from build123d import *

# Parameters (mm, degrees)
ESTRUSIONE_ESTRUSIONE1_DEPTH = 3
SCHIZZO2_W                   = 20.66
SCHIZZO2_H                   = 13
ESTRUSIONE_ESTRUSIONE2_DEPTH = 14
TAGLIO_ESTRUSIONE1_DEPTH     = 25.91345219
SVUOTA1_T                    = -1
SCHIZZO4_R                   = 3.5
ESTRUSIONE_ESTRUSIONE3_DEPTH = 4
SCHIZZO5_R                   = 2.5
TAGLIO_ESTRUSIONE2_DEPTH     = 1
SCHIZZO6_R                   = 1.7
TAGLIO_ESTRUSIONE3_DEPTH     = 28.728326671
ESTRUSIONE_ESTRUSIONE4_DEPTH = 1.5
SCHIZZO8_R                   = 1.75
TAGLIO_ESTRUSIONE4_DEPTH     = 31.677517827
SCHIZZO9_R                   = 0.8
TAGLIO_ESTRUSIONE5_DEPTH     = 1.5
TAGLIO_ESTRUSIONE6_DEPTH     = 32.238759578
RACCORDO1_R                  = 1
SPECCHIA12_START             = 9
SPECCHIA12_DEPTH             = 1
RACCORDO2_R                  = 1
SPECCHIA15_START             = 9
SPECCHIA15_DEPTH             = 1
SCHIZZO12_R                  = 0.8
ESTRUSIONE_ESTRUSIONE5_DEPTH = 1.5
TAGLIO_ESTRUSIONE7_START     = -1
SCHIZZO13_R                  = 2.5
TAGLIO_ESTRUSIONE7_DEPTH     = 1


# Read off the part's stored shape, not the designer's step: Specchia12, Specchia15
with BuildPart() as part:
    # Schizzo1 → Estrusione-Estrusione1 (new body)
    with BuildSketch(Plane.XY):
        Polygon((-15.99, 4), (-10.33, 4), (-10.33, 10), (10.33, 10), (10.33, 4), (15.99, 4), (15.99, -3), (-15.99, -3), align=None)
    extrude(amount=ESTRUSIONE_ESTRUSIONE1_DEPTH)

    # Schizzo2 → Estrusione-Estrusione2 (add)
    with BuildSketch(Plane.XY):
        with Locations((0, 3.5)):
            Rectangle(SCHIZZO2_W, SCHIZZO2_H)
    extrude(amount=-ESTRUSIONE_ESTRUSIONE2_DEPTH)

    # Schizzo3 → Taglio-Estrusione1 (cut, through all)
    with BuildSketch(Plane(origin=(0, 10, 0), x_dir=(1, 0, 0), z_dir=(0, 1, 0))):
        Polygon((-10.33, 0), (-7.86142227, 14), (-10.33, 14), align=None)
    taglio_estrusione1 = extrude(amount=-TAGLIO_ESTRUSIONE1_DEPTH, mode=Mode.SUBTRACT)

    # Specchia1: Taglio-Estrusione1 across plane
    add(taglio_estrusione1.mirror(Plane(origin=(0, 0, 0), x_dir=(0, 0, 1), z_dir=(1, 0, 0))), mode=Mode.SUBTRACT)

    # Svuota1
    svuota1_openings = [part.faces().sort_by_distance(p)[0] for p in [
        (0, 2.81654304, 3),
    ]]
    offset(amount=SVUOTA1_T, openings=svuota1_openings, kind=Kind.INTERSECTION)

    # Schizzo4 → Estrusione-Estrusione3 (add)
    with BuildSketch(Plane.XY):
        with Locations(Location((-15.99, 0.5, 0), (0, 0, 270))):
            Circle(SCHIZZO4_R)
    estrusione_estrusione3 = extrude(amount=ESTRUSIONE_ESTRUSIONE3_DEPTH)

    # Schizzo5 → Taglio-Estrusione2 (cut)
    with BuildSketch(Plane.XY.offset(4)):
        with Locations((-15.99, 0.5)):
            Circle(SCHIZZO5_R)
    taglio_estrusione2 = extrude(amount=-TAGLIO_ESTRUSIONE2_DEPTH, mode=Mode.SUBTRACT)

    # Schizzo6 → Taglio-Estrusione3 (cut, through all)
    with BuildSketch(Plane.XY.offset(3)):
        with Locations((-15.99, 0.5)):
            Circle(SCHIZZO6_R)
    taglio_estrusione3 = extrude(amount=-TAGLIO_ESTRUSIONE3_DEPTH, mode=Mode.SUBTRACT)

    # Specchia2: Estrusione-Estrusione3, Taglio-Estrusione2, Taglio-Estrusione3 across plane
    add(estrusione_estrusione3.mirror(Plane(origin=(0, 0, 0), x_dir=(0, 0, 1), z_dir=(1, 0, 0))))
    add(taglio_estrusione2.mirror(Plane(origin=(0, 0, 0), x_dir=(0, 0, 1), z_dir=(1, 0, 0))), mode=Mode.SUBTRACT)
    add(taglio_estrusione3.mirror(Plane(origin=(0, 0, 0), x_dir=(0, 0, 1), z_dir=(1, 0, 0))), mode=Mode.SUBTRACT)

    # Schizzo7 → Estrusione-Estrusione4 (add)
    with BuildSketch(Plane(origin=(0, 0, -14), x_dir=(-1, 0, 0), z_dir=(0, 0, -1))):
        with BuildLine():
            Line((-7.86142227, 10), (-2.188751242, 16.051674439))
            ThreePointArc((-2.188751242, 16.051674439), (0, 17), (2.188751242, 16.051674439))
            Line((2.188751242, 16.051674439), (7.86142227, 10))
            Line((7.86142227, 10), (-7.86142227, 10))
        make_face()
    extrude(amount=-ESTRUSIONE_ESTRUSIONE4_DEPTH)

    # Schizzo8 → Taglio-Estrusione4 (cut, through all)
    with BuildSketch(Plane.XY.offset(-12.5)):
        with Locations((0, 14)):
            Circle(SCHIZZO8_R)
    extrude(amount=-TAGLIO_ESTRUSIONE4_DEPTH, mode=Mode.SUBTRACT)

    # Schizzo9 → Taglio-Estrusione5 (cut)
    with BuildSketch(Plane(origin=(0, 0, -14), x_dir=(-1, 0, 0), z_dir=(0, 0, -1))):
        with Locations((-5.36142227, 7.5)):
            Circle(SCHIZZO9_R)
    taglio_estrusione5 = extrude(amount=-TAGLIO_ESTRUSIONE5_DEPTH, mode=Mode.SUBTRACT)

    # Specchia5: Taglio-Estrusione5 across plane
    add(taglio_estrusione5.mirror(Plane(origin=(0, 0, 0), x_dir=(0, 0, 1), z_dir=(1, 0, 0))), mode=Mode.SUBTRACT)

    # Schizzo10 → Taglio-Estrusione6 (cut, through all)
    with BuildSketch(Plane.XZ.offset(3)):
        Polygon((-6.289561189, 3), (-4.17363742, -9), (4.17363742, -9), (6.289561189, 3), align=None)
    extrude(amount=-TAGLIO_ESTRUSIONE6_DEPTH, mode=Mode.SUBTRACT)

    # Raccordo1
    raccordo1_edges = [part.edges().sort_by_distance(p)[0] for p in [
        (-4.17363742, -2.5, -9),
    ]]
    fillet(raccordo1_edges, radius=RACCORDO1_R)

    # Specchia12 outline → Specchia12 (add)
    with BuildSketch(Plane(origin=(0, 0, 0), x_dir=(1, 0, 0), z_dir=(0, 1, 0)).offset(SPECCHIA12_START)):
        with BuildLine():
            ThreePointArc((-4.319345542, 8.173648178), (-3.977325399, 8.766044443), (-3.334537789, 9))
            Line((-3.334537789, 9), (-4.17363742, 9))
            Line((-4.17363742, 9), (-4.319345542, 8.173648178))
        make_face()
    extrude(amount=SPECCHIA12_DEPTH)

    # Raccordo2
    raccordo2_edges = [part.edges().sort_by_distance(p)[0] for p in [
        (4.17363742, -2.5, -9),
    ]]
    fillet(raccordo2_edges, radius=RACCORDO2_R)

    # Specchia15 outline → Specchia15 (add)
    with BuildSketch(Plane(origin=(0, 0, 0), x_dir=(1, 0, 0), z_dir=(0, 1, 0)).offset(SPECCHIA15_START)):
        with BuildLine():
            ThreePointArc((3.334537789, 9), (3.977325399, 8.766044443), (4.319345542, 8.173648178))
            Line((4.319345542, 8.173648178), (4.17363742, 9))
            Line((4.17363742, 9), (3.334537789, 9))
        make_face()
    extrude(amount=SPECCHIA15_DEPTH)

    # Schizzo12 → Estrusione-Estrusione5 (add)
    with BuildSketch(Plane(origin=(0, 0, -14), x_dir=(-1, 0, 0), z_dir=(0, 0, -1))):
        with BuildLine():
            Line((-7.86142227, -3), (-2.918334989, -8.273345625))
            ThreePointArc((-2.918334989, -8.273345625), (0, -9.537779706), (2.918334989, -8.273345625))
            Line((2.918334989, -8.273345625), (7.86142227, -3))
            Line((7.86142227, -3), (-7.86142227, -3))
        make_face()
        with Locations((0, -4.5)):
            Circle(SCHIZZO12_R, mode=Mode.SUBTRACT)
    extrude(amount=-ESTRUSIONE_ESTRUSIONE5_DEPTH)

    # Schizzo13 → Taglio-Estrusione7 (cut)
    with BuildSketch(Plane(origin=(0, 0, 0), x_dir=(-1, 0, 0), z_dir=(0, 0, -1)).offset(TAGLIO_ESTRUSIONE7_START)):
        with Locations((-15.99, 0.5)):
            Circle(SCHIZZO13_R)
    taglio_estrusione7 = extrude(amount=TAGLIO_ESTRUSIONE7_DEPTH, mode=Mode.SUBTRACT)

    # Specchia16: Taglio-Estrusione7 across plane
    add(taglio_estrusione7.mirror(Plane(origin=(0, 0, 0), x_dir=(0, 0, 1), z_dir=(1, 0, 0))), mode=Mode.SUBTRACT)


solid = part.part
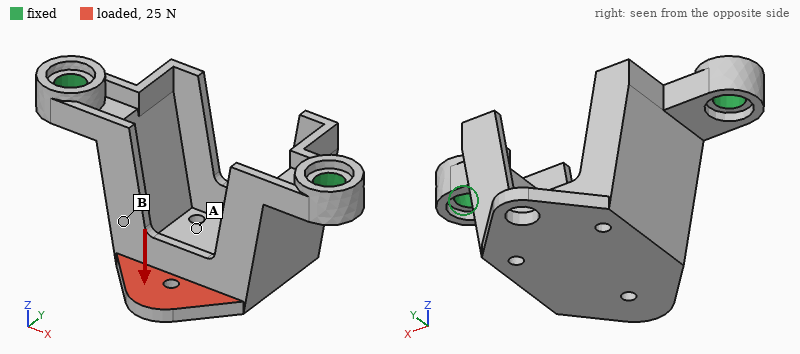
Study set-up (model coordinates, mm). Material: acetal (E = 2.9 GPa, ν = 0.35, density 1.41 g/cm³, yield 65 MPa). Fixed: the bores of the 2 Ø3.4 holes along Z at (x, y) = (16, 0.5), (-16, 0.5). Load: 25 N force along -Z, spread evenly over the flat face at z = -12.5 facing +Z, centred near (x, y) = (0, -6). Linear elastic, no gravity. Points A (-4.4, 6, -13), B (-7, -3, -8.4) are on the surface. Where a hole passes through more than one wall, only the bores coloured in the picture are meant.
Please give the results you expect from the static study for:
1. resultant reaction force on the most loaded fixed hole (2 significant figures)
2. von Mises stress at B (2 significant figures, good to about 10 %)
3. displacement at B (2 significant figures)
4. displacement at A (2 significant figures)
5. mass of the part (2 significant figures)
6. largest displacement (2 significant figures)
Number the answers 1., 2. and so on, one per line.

1. 15 N
2. 4.3 MPa
3. 0.19 mm
4. 0.28 mm
5. 1.9 g
6. 0.53 mm
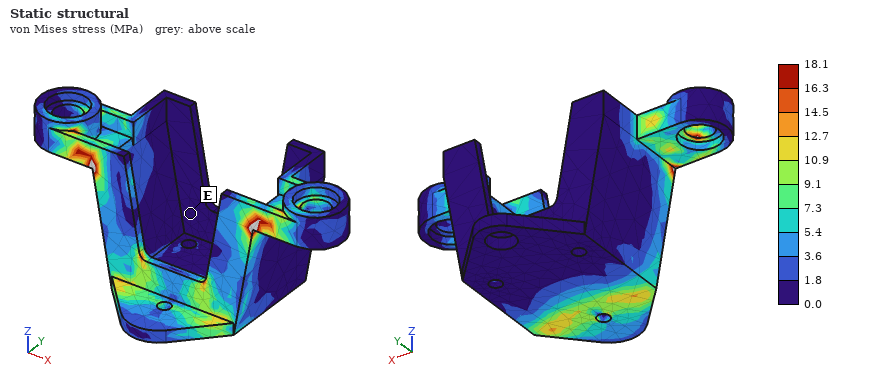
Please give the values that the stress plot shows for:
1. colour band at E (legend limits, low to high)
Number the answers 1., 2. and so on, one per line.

1. 0.0 to 1.8 MPa
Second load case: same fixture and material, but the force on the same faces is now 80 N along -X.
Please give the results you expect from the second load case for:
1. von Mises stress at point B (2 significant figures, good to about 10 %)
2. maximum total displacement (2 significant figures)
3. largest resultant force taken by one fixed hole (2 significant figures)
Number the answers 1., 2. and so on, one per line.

1. 9.7 MPa
2. 0.51 mm
3. 61 N
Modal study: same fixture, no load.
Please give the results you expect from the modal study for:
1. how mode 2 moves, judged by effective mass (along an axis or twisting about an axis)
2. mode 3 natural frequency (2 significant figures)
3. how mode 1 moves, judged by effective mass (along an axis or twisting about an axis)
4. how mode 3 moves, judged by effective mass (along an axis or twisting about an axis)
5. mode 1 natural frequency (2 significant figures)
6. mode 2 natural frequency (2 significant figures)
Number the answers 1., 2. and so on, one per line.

1. along X
2. 3200 Hz
3. along Y
4. along X
5. 920 Hz
6. 1900 Hz
